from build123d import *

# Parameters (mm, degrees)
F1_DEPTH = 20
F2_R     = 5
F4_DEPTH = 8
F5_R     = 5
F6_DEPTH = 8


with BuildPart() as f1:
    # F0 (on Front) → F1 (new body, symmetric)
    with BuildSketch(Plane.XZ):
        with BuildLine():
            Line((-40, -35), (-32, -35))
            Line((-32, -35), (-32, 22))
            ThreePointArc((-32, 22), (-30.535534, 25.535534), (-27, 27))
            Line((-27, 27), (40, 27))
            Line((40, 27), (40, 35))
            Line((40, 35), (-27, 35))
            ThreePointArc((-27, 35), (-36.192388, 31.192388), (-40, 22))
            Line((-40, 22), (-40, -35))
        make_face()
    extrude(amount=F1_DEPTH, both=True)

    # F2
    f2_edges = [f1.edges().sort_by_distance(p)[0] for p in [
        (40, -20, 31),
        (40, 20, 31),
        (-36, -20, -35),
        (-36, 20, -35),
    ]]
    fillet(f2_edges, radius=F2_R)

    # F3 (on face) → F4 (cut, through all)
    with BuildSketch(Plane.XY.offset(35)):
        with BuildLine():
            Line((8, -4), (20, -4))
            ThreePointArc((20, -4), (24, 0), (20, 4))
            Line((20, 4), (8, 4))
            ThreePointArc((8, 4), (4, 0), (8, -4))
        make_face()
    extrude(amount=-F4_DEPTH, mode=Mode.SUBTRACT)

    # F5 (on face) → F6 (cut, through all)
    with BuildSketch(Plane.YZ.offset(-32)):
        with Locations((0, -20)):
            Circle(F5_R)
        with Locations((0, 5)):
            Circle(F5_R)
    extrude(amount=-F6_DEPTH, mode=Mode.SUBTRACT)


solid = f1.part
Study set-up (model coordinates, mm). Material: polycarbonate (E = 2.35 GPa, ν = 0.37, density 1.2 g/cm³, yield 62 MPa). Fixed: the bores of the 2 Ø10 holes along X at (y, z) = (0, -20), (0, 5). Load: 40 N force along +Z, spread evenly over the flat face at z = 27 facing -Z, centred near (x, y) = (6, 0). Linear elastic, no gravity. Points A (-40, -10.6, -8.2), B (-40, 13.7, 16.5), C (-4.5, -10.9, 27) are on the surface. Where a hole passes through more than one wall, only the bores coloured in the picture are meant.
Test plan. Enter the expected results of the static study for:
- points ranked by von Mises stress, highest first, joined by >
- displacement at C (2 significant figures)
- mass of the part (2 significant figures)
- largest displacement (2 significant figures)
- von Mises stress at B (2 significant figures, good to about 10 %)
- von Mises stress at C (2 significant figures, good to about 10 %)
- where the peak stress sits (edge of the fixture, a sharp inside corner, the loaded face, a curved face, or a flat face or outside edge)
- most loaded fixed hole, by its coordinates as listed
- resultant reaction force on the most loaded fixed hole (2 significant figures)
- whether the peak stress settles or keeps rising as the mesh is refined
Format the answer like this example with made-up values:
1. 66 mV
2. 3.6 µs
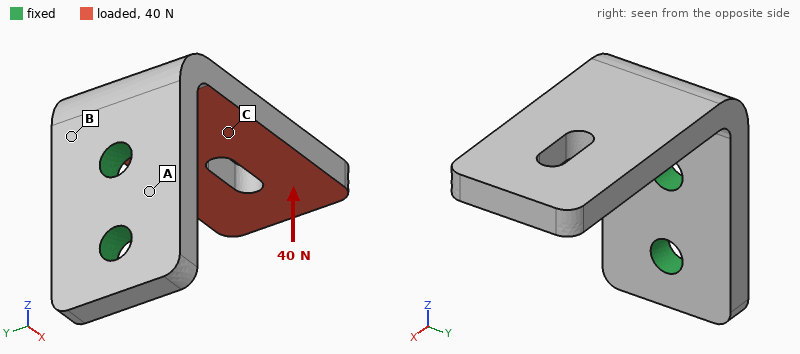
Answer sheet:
1. B > C > A
2. 0.41 mm
3. 50 g
4. 1.2 mm
5. 3.3 MPa
6. 1.4 MPa
7. edge of the fixture
8. (0, 5)
9. 39 N
10. keeps rising
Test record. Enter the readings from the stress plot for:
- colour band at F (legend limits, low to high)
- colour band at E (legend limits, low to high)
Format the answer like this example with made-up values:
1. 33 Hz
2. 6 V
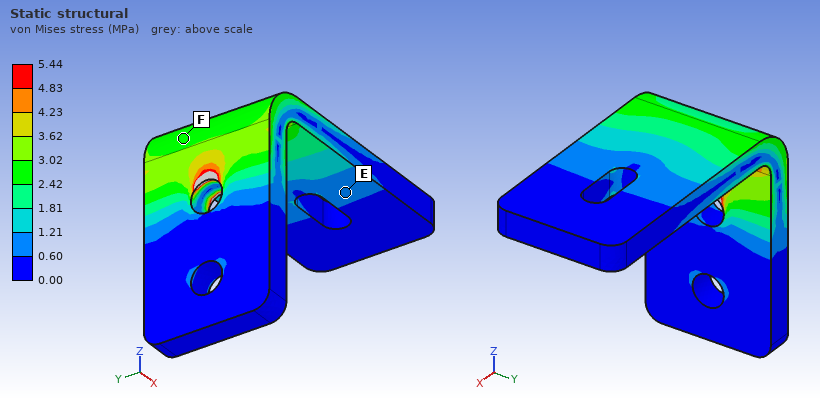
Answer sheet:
1. 2.42 to 3.02 MPa
2. 0.60 to 1.21 MPa
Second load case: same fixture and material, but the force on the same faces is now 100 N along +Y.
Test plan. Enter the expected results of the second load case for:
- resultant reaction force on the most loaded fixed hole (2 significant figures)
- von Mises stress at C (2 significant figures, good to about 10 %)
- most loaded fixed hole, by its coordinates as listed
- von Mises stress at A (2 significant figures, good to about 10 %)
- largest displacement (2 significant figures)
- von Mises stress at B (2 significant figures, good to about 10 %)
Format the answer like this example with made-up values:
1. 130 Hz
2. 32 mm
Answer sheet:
1. 140 N
2. 1.3 MPa
3. (0, 5)
4. 1.9 MPa
5. 1.2 mm
6. 4.8 MPa
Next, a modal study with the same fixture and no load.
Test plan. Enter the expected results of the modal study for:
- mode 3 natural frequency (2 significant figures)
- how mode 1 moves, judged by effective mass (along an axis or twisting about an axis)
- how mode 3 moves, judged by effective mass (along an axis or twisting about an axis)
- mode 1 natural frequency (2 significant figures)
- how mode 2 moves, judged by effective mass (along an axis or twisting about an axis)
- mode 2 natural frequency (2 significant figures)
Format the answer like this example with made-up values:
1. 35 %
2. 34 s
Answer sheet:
1. 1000 Hz
2. along Z
3. along X
4. 230 Hz
5. along Y
6. 350 Hz
